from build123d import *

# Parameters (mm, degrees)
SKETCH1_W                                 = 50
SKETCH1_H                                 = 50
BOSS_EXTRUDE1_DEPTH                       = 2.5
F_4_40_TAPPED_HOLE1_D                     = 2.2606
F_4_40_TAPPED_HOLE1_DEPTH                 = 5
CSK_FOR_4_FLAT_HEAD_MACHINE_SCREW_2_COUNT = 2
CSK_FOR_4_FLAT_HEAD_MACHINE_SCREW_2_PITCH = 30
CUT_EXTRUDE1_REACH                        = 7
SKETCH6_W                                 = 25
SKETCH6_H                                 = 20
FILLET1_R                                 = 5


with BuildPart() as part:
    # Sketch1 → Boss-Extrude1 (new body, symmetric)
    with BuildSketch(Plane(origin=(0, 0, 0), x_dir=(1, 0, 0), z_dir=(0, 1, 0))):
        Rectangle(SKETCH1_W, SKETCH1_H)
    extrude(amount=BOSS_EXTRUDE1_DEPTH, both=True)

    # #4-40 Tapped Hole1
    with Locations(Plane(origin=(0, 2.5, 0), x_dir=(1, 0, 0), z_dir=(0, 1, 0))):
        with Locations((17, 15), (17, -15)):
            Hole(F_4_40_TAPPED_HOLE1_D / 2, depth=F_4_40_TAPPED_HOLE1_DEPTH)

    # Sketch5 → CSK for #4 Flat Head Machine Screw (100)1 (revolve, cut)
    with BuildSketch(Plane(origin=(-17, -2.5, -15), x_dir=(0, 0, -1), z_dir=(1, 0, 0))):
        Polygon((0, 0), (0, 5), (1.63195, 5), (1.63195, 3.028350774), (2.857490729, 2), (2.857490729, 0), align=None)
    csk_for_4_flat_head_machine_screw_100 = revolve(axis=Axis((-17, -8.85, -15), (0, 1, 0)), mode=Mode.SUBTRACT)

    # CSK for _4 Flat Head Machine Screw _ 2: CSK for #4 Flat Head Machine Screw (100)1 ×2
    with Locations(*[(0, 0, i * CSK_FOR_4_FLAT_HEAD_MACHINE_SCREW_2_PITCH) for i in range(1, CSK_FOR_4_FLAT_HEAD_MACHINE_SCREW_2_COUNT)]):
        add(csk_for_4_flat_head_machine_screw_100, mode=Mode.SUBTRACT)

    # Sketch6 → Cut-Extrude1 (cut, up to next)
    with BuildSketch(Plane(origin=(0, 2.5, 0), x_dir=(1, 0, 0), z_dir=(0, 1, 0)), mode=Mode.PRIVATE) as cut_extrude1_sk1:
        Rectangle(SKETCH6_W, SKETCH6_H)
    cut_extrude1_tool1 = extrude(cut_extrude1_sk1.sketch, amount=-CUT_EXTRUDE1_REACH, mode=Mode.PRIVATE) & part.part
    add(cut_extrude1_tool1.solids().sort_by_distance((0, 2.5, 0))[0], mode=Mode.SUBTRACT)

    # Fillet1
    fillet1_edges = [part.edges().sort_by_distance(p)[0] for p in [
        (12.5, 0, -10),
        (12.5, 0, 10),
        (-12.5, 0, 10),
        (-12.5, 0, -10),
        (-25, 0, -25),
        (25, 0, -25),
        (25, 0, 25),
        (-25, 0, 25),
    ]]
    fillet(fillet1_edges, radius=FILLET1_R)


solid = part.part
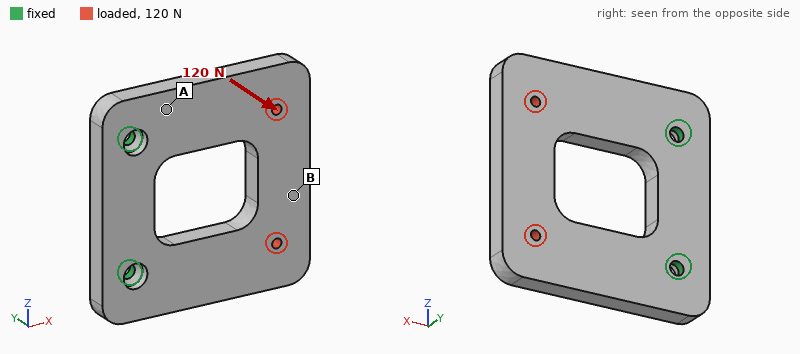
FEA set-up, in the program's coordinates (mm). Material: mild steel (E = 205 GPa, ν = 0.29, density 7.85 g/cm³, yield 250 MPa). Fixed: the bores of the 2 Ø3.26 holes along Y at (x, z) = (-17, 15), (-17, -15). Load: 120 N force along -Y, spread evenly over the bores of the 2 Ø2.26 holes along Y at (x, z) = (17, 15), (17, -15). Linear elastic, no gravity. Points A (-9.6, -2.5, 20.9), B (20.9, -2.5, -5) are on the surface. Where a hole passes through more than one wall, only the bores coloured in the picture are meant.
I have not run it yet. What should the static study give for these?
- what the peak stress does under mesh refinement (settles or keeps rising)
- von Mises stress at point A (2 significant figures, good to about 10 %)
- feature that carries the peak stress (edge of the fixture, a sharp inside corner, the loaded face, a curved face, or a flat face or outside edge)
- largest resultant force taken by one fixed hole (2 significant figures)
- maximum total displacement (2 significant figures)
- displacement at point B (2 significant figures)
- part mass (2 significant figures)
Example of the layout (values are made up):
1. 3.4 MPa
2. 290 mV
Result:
1. keeps rising
2. 24 MPa
3. edge of the fixture
4. 60 N
5. 58 µm
6. 52 µm
7. 77 g
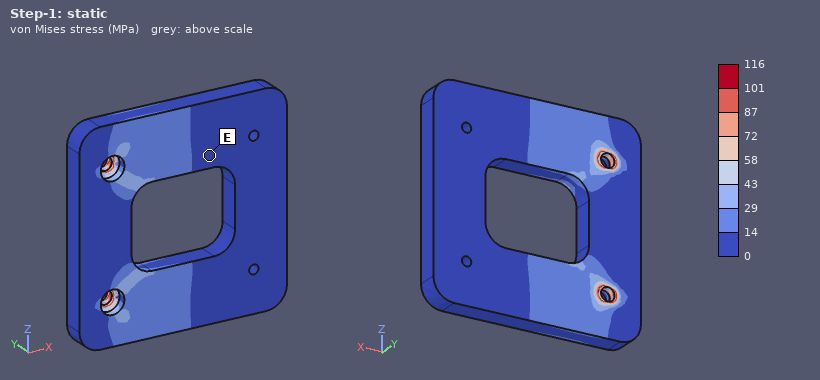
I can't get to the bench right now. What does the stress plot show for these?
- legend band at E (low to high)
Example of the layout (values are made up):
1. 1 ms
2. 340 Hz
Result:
1. 0 to 14 MPa
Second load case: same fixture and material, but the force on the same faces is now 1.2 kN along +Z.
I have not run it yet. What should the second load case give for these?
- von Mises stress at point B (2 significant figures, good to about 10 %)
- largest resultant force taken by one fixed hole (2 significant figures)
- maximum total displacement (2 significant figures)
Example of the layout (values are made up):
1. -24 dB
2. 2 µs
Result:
1. 19 MPa
2. 1.4 kN
3. 24 µm
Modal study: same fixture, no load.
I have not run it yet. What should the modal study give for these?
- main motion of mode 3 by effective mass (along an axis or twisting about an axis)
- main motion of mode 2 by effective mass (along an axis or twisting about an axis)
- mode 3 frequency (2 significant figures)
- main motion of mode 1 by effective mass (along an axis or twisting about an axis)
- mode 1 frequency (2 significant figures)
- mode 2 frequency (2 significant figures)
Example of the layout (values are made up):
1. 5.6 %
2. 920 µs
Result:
1. along Z
2. twisting about X
3. 6500 Hz
4. along Y
5. 1400 Hz
6. 3500 Hz
